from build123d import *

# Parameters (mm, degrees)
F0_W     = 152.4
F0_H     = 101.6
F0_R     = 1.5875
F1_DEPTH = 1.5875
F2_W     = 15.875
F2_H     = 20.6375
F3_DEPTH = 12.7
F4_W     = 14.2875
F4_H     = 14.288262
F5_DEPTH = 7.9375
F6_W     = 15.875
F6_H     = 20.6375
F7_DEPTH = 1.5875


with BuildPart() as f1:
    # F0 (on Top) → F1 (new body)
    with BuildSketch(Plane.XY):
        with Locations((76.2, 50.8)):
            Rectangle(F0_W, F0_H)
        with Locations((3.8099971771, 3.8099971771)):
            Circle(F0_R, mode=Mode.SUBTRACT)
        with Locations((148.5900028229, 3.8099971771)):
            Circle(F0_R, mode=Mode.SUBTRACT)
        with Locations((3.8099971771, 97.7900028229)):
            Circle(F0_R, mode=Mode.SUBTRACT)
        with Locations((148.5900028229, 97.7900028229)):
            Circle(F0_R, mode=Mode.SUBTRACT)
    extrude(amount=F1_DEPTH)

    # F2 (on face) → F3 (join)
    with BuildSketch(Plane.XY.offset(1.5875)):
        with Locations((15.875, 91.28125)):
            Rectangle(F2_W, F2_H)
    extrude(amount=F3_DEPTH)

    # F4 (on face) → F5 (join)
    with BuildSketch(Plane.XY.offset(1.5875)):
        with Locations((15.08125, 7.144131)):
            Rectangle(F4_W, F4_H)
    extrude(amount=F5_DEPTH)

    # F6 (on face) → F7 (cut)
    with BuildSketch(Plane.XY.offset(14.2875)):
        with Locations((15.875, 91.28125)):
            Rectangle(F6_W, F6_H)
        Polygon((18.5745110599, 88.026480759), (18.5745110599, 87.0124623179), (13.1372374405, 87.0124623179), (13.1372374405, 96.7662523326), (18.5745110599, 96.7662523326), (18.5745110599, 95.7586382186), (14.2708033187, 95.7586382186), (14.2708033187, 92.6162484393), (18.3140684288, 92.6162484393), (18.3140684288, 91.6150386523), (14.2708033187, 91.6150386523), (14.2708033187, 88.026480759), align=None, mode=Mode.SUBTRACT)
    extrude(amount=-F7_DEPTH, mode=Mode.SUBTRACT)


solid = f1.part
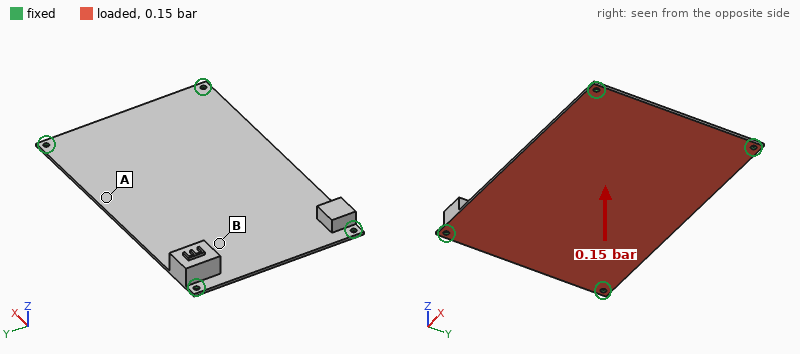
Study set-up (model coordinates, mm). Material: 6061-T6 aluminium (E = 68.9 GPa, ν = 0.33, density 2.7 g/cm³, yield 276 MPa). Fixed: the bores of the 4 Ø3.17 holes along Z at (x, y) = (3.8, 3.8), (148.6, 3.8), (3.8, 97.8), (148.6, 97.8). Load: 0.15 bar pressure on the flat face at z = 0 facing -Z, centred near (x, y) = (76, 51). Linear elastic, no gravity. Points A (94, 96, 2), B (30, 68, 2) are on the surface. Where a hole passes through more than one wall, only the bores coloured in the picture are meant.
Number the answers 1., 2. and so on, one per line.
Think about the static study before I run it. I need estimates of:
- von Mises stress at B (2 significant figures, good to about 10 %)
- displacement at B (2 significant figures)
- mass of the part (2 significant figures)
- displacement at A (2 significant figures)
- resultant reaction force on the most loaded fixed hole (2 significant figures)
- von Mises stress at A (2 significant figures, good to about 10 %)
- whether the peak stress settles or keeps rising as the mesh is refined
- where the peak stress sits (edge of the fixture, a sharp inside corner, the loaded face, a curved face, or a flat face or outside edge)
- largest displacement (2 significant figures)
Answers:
1. 12 MPa
2. 0.60 mm
3. 81 g
4. 1.0 mm
5. 66 N
6. 38 MPa
7. keeps rising
8. edge of the fixture
9. 1.2 mm
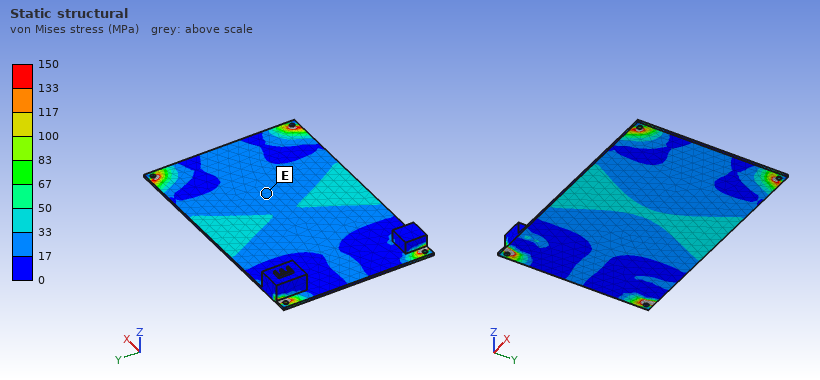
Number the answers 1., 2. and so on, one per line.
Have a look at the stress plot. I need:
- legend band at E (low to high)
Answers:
1. 17 to 33 MPa
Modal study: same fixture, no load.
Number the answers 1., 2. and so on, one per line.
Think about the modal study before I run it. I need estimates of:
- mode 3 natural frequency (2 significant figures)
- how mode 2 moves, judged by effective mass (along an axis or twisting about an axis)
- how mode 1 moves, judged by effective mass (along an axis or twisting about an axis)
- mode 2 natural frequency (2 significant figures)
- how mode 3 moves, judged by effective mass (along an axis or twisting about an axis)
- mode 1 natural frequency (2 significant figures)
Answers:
1. 760 Hz
2. twisting about X
3. along Z
4. 560 Hz
5. twisting about Y
6. 310 Hz
